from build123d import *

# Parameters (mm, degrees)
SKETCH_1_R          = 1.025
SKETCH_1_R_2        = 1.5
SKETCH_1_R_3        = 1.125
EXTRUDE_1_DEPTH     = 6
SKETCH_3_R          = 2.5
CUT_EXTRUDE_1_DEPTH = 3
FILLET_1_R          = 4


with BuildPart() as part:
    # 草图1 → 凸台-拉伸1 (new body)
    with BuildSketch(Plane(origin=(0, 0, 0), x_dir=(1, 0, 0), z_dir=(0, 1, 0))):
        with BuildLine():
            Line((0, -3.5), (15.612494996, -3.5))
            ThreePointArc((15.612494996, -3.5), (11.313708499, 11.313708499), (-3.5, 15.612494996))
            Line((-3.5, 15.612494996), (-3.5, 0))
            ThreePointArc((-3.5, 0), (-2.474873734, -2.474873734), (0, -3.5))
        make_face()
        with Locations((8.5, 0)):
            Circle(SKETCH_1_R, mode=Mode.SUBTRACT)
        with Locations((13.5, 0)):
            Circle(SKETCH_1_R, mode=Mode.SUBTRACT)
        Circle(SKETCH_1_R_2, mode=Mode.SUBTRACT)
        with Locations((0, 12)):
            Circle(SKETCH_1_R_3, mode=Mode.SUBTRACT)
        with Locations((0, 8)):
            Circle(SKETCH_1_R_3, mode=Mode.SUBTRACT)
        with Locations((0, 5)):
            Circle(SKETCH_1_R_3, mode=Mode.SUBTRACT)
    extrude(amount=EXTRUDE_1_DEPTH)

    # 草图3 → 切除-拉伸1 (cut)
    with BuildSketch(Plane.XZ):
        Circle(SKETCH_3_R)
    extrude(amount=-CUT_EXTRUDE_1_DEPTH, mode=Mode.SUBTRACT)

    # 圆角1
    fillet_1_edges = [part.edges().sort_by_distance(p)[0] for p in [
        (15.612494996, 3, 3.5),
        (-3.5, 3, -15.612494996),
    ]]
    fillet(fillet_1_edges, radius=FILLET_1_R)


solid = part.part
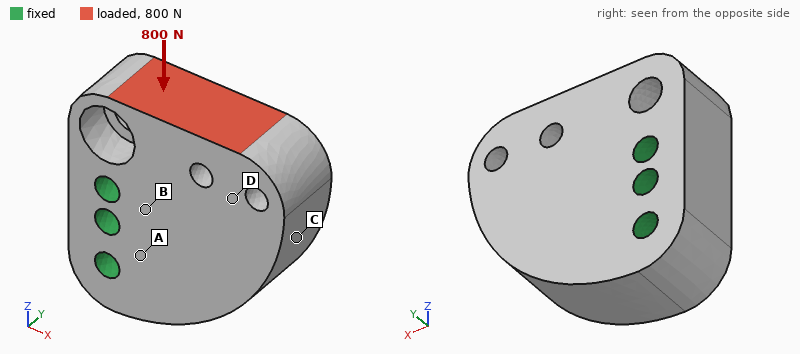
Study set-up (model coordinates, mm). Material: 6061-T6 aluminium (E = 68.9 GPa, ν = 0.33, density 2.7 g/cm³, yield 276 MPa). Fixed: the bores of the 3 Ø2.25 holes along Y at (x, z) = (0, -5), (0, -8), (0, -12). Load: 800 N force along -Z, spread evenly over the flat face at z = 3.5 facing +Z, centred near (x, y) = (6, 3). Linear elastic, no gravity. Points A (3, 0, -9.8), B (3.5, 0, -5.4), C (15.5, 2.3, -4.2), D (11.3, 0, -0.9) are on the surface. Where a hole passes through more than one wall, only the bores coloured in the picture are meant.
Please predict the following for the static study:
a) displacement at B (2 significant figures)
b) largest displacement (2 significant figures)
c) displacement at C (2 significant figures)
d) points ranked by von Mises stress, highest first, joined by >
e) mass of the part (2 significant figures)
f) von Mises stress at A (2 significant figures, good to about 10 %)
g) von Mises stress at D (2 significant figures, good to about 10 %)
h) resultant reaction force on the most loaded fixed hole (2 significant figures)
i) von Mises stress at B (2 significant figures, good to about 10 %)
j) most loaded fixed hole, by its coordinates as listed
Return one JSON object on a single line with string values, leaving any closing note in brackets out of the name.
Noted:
{"displacement at B": "1.8 µm", "largest displacement": "8.1 µm", "displacement at C": "7.2 µm", "points ranked by von Mises stress, highest first, joined by >": "B > A > D > C", "mass of the part": "4.6 g", "von Mises stress at A": "19 MPa", "von Mises stress at D": "9.1 MPa", "resultant reaction force on the most loaded fixed hole": "610 N", "von Mises stress at B": "26 MPa", "most loaded fixed hole, by its coordinates as listed": "(0, -5)"}
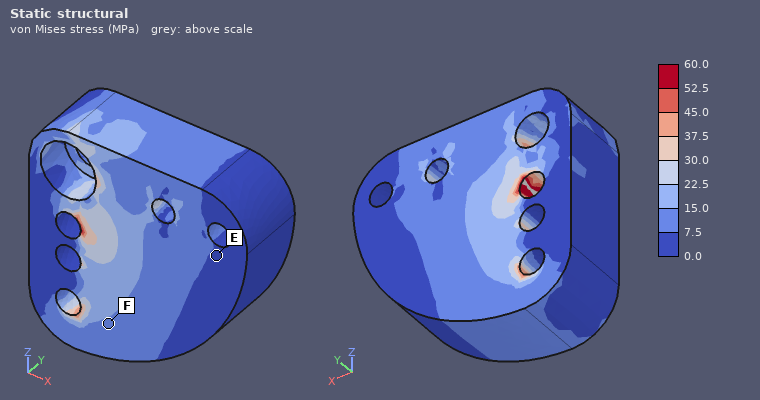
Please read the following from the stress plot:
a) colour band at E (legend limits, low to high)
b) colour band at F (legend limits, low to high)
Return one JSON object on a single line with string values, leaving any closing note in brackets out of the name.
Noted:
{"colour band at E": "0.0 to 7.5 MPa", "colour band at F": "7.5 to 15.0 MPa"}
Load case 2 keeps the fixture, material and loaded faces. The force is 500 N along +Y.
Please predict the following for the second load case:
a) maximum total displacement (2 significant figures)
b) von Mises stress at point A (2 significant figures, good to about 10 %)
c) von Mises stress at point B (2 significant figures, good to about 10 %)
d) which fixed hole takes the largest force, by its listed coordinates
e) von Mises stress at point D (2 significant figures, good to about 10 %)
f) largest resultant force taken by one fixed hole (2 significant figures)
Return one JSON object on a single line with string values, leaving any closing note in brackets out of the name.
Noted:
{"maximum total displacement": "26 µm", "von Mises stress at point A": "29 MPa", "von Mises stress at point B": "49 MPa", "which fixed hole takes the largest force, by its listed coordinates": "(0, -5)", "von Mises stress at point D": "20 MPa", "largest resultant force taken by one fixed hole": "620 N"}
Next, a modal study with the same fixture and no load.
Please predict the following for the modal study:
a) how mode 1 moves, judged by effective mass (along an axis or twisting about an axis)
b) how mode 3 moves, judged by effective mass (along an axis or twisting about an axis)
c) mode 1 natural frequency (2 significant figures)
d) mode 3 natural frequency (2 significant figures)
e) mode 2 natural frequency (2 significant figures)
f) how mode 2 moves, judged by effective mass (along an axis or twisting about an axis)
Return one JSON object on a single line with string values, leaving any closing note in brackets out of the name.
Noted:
{"how mode 1 moves, judged by effective mass": "along Y", "how mode 3 moves, judged by effective mass": "twisting about X", "mode 1 natural frequency": "19 kHz", "mode 3 natural frequency": "37 kHz", "mode 2 natural frequency": "28 kHz", "how mode 2 moves, judged by effective mass": "along Z"}
